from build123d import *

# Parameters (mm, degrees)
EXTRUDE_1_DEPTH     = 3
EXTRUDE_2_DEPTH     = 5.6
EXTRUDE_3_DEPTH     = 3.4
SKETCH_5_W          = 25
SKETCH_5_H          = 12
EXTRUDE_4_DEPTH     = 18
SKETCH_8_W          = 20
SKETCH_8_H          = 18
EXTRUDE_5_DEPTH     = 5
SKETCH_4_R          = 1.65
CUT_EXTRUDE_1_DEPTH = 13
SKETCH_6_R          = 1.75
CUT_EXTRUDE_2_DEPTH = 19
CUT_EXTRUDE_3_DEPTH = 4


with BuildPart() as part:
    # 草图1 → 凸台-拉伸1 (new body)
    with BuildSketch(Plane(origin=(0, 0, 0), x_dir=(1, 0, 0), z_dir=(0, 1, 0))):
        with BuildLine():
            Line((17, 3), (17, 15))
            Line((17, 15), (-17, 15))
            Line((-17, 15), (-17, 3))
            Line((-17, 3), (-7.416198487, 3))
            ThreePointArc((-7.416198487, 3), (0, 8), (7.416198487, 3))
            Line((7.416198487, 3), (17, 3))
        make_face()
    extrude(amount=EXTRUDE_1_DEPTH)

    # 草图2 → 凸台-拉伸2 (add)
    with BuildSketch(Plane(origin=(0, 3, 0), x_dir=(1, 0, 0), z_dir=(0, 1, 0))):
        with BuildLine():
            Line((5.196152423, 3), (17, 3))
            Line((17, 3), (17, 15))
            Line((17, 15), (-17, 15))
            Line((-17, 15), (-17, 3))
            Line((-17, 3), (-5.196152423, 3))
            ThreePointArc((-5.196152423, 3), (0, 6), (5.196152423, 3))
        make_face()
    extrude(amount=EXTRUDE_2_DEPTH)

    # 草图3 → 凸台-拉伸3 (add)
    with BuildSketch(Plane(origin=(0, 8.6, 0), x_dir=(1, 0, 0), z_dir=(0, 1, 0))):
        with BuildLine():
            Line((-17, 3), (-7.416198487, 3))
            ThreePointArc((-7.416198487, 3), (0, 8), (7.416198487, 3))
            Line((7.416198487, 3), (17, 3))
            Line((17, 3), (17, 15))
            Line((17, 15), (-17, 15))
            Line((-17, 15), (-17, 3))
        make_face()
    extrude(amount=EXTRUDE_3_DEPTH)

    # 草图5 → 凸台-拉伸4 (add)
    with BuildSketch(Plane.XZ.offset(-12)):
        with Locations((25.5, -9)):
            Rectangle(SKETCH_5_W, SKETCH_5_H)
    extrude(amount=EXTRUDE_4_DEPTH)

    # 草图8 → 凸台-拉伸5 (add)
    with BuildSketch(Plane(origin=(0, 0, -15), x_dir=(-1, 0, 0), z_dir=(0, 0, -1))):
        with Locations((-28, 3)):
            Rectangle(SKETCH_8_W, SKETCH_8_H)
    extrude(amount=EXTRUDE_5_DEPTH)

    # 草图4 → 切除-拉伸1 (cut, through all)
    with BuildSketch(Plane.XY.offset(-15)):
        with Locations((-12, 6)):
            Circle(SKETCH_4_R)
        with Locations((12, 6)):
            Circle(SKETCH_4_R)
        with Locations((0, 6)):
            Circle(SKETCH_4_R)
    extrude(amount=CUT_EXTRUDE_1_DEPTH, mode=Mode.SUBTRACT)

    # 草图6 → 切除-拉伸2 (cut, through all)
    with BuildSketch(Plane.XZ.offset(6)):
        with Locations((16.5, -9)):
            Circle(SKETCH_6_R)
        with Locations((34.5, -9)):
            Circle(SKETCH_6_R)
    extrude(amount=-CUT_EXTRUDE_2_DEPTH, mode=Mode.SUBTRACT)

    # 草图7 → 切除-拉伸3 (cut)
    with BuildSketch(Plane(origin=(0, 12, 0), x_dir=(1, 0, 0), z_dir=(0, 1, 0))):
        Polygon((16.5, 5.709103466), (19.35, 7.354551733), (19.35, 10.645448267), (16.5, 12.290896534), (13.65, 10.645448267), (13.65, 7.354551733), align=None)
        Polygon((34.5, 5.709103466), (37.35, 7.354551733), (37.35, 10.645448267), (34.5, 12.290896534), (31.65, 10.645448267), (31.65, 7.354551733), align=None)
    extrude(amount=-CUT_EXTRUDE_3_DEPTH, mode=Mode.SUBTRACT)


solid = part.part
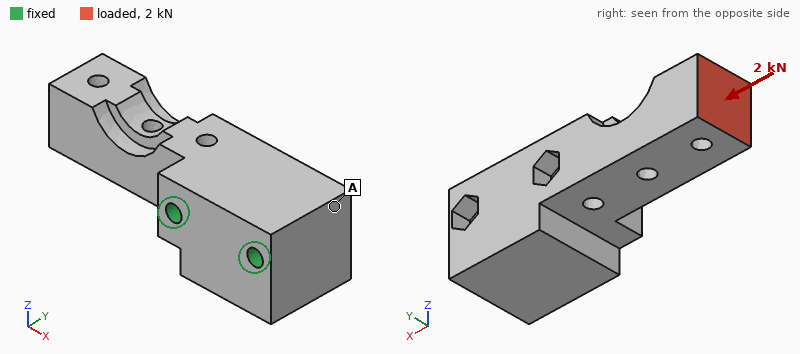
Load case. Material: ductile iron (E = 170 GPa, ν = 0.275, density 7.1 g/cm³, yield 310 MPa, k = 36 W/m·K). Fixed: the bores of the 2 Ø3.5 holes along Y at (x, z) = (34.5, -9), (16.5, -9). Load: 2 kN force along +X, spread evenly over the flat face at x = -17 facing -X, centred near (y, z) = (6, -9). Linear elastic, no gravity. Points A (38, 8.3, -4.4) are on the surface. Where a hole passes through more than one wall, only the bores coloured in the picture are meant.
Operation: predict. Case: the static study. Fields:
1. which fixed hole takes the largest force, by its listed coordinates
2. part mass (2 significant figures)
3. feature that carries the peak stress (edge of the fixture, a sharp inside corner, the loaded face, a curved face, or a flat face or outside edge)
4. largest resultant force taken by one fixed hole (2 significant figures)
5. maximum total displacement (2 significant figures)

(16.5, -9)
73 g
a curved face
1.6 kN
15 µm
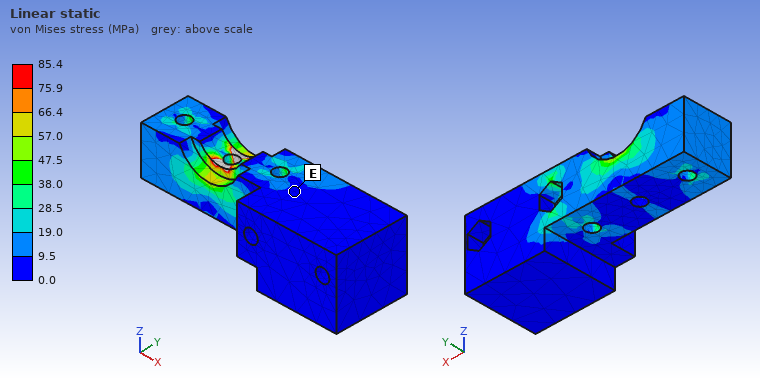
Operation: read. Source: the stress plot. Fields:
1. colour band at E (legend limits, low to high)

0.0 to 9.5 MPa
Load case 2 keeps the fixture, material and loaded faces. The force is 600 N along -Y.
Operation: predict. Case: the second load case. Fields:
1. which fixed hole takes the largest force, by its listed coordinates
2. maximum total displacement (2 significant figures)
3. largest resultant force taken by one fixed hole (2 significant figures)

(16.5, -9)
46 µm
1.2 kN
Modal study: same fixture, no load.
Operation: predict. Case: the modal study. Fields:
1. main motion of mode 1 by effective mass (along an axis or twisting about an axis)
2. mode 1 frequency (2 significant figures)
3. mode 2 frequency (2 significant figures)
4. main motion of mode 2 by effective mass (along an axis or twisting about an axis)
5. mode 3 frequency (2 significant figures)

along Z
5800 Hz
6600 Hz
along Y
17 kHz
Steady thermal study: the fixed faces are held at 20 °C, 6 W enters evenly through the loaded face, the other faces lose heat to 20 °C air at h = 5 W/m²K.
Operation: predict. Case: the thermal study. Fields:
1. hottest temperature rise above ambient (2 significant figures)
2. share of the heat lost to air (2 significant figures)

52 K
4.3 %
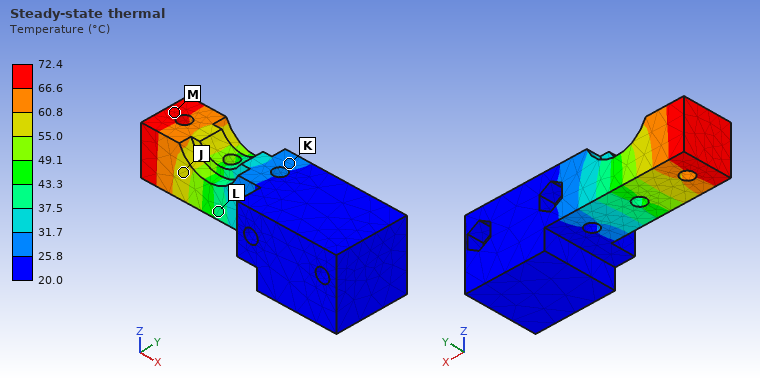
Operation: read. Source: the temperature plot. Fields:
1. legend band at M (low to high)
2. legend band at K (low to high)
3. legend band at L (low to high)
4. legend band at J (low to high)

66.6 to 72.4 °C
25.8 to 31.7 °C
37.5 to 43.3 °C
55.0 to 60.8 °C
